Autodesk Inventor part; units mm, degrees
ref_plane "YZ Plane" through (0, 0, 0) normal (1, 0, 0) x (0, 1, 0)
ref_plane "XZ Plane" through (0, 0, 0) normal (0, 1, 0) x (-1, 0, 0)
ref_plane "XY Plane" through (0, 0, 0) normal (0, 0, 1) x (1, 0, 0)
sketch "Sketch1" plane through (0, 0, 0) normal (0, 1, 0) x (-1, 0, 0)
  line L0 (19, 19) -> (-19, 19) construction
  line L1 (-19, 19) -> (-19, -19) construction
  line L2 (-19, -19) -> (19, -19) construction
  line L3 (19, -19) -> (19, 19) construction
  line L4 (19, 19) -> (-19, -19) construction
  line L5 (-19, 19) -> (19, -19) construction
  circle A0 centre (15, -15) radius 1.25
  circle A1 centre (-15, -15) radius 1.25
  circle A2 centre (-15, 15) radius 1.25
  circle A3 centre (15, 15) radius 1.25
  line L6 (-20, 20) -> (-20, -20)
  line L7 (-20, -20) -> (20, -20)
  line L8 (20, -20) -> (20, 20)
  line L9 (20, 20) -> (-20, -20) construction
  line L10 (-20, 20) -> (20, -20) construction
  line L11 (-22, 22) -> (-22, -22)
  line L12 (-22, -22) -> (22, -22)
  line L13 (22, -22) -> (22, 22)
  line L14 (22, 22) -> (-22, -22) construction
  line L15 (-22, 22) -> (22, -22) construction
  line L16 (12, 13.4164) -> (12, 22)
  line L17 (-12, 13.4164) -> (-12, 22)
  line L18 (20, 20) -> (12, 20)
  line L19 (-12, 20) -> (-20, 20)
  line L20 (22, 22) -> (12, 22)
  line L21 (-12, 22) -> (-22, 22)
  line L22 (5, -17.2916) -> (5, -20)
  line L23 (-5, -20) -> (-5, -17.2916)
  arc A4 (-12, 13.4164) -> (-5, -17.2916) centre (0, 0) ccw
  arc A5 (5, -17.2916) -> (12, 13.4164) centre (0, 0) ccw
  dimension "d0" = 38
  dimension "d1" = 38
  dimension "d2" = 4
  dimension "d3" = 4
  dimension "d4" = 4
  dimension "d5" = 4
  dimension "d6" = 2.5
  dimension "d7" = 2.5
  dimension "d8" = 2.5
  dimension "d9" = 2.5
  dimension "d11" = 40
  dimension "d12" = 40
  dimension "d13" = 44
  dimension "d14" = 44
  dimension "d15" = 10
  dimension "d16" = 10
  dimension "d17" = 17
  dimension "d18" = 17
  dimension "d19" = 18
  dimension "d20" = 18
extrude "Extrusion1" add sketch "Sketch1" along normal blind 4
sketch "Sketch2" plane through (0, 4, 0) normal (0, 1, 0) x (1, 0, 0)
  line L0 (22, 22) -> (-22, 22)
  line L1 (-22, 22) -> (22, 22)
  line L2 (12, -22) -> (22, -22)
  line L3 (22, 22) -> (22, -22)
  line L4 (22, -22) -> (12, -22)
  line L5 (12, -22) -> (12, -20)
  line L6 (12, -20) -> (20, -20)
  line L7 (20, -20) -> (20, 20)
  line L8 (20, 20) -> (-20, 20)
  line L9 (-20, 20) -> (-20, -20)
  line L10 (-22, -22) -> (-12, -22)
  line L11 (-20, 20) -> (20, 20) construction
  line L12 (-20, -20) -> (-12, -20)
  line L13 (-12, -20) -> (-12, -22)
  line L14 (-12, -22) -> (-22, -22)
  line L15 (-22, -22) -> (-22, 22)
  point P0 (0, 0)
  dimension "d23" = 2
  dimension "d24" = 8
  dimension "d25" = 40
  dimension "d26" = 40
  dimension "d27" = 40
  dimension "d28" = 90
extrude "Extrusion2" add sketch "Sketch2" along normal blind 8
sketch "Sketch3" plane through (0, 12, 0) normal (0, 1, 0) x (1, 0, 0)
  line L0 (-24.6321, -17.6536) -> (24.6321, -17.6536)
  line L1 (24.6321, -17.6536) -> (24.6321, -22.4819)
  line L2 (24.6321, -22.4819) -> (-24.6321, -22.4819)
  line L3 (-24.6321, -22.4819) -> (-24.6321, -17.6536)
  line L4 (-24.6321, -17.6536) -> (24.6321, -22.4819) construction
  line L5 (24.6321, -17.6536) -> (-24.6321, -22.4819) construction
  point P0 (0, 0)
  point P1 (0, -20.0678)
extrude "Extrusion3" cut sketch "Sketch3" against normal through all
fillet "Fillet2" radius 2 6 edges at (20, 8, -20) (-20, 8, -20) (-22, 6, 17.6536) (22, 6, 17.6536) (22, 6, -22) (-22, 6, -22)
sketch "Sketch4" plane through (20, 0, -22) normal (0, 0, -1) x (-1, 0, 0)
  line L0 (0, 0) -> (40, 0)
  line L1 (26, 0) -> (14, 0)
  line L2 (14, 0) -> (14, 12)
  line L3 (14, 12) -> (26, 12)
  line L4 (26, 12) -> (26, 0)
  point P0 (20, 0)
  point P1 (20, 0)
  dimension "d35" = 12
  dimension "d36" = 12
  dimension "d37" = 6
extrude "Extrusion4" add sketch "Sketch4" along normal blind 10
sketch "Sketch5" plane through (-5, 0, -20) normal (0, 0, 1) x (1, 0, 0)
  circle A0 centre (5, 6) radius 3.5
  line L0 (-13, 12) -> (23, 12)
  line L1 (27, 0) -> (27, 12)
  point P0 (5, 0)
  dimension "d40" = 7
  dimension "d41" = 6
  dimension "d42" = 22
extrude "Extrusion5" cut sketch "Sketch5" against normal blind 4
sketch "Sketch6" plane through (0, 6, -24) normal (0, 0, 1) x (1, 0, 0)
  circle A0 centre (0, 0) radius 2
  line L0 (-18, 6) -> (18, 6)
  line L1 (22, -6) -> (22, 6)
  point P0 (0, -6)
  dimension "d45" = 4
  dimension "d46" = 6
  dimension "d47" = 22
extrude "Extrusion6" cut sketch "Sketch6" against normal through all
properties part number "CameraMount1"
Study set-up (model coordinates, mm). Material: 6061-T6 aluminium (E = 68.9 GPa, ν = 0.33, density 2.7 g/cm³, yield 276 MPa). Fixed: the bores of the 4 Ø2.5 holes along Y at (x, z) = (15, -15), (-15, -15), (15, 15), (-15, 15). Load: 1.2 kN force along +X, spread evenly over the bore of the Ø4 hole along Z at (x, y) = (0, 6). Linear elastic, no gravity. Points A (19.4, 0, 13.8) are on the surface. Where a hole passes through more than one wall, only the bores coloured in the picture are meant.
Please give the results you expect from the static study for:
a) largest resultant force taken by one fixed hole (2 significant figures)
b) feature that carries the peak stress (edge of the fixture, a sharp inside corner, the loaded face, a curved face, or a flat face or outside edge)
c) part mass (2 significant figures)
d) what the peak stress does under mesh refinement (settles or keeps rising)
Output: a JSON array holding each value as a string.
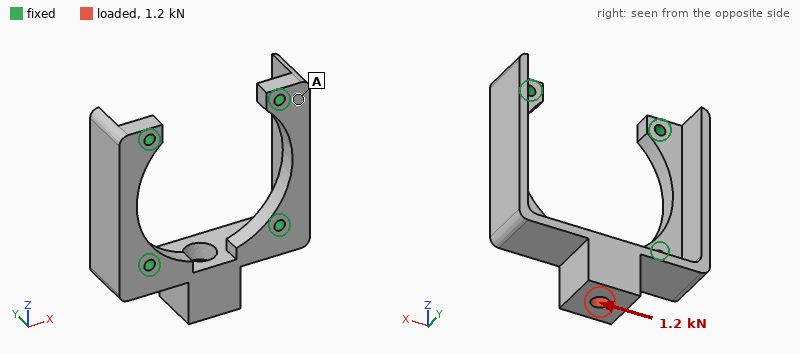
["850 N", "edge of the fixture", "15 g", "keeps rising"]
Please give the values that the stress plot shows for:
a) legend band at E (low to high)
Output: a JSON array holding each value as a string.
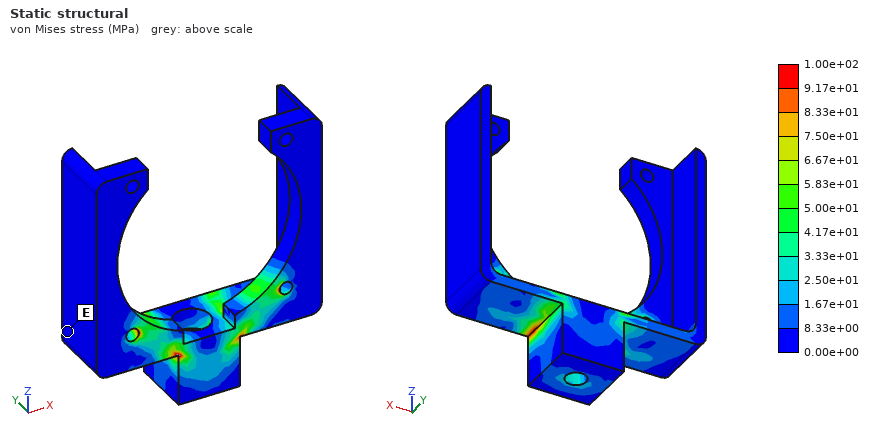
["0.00e+00 to 8.33e+00 MPa"]
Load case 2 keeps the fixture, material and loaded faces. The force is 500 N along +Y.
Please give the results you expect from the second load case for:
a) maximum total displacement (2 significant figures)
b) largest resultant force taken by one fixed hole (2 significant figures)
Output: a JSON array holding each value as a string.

["0.14 mm", "320 N"]
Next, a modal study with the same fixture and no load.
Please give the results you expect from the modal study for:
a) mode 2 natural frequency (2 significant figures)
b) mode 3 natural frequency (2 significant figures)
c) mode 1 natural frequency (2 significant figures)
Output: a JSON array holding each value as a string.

["13 kHz", "14 kHz", "5800 Hz"]
